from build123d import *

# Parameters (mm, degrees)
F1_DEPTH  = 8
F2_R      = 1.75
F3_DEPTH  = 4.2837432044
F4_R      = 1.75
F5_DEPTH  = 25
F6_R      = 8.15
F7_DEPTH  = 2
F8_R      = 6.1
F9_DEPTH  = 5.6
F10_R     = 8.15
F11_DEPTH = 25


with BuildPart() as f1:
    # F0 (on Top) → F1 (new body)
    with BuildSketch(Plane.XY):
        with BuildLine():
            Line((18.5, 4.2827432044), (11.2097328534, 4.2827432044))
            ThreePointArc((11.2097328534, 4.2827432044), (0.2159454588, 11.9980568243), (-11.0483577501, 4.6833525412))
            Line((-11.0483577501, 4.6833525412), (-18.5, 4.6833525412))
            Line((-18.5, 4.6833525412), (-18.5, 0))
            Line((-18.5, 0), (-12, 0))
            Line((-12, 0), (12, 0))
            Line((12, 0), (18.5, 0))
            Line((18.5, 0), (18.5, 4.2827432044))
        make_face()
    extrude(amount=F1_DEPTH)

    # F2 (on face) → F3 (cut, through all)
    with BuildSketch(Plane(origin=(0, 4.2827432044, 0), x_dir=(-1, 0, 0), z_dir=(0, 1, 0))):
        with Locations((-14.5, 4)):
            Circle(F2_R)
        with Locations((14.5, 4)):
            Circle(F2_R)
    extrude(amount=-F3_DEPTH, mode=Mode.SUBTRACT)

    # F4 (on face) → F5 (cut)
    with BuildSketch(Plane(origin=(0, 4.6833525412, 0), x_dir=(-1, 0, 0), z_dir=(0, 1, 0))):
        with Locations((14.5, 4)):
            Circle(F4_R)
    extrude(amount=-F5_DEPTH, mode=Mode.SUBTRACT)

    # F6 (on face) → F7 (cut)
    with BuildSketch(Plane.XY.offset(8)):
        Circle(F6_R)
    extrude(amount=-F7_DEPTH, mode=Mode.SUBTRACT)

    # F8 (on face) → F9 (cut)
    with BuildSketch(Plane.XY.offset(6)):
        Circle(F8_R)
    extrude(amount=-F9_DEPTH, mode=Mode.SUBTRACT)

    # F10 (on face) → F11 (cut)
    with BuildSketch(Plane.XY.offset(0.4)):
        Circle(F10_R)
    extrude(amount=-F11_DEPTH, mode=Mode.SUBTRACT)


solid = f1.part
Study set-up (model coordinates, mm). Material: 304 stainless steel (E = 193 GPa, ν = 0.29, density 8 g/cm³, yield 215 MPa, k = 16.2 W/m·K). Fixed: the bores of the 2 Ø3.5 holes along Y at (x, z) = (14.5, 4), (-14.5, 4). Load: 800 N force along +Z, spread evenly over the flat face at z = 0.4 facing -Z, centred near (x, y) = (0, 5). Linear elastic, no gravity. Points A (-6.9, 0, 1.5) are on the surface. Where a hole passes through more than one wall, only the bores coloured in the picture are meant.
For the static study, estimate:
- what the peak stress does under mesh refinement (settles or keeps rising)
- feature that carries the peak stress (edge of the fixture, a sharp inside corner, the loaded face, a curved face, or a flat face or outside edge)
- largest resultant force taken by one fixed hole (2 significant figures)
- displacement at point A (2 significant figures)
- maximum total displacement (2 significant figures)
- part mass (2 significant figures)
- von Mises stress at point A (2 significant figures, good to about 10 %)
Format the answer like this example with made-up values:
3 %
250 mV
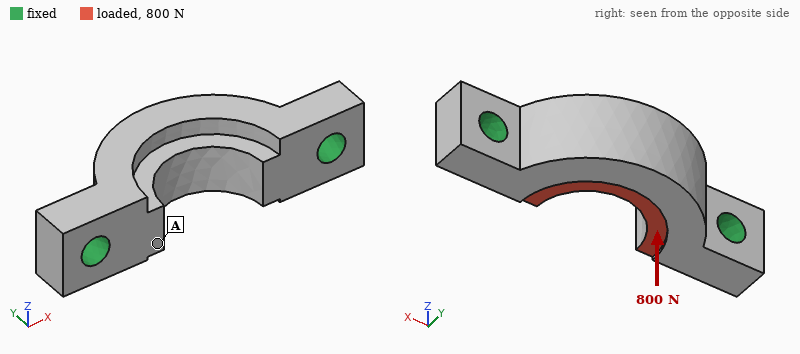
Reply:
keeps rising
edge of the fixture
410 N
2.3 µm
6.7 µm
13 g
17 MPa
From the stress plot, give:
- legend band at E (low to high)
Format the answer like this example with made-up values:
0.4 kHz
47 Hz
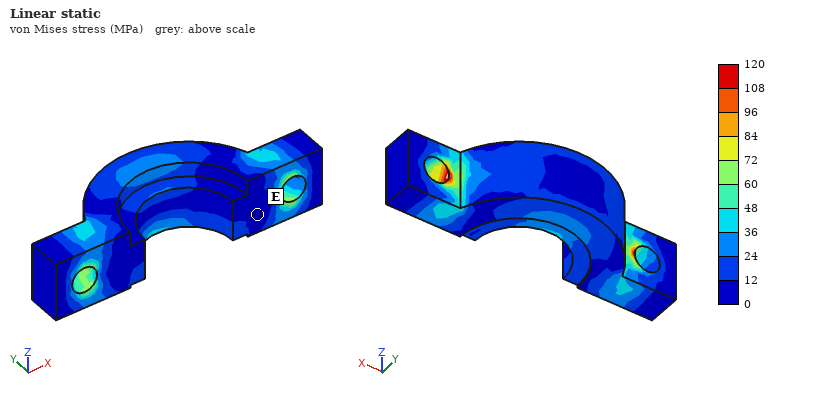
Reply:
0 to 12 MPa
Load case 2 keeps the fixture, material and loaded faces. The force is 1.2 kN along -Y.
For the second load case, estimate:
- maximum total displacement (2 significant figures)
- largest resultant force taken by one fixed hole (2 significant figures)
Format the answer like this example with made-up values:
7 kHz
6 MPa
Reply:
11 µm
780 N
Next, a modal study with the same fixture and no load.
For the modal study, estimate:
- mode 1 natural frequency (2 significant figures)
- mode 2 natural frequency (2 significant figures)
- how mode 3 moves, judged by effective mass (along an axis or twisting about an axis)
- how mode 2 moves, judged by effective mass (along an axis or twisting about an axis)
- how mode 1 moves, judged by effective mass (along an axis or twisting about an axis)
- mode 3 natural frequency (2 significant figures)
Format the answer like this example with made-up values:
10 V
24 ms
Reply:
19 kHz
38 kHz
along X
along Y
along Z
48 kHz
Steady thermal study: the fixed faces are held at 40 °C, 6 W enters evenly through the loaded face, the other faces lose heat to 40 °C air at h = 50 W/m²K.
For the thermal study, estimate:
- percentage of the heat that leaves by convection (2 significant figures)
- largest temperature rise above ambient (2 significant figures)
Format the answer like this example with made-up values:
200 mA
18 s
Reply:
17 %
49 K
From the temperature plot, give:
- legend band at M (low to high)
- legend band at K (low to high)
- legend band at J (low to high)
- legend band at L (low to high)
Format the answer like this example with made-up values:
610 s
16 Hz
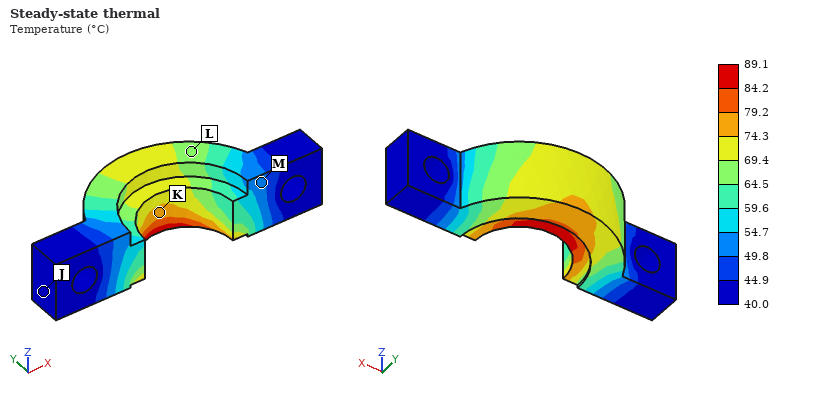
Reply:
49.8 to 54.7 °C
74.3 to 79.2 °C
40.0 to 44.9 °C
64.5 to 69.4 °C
